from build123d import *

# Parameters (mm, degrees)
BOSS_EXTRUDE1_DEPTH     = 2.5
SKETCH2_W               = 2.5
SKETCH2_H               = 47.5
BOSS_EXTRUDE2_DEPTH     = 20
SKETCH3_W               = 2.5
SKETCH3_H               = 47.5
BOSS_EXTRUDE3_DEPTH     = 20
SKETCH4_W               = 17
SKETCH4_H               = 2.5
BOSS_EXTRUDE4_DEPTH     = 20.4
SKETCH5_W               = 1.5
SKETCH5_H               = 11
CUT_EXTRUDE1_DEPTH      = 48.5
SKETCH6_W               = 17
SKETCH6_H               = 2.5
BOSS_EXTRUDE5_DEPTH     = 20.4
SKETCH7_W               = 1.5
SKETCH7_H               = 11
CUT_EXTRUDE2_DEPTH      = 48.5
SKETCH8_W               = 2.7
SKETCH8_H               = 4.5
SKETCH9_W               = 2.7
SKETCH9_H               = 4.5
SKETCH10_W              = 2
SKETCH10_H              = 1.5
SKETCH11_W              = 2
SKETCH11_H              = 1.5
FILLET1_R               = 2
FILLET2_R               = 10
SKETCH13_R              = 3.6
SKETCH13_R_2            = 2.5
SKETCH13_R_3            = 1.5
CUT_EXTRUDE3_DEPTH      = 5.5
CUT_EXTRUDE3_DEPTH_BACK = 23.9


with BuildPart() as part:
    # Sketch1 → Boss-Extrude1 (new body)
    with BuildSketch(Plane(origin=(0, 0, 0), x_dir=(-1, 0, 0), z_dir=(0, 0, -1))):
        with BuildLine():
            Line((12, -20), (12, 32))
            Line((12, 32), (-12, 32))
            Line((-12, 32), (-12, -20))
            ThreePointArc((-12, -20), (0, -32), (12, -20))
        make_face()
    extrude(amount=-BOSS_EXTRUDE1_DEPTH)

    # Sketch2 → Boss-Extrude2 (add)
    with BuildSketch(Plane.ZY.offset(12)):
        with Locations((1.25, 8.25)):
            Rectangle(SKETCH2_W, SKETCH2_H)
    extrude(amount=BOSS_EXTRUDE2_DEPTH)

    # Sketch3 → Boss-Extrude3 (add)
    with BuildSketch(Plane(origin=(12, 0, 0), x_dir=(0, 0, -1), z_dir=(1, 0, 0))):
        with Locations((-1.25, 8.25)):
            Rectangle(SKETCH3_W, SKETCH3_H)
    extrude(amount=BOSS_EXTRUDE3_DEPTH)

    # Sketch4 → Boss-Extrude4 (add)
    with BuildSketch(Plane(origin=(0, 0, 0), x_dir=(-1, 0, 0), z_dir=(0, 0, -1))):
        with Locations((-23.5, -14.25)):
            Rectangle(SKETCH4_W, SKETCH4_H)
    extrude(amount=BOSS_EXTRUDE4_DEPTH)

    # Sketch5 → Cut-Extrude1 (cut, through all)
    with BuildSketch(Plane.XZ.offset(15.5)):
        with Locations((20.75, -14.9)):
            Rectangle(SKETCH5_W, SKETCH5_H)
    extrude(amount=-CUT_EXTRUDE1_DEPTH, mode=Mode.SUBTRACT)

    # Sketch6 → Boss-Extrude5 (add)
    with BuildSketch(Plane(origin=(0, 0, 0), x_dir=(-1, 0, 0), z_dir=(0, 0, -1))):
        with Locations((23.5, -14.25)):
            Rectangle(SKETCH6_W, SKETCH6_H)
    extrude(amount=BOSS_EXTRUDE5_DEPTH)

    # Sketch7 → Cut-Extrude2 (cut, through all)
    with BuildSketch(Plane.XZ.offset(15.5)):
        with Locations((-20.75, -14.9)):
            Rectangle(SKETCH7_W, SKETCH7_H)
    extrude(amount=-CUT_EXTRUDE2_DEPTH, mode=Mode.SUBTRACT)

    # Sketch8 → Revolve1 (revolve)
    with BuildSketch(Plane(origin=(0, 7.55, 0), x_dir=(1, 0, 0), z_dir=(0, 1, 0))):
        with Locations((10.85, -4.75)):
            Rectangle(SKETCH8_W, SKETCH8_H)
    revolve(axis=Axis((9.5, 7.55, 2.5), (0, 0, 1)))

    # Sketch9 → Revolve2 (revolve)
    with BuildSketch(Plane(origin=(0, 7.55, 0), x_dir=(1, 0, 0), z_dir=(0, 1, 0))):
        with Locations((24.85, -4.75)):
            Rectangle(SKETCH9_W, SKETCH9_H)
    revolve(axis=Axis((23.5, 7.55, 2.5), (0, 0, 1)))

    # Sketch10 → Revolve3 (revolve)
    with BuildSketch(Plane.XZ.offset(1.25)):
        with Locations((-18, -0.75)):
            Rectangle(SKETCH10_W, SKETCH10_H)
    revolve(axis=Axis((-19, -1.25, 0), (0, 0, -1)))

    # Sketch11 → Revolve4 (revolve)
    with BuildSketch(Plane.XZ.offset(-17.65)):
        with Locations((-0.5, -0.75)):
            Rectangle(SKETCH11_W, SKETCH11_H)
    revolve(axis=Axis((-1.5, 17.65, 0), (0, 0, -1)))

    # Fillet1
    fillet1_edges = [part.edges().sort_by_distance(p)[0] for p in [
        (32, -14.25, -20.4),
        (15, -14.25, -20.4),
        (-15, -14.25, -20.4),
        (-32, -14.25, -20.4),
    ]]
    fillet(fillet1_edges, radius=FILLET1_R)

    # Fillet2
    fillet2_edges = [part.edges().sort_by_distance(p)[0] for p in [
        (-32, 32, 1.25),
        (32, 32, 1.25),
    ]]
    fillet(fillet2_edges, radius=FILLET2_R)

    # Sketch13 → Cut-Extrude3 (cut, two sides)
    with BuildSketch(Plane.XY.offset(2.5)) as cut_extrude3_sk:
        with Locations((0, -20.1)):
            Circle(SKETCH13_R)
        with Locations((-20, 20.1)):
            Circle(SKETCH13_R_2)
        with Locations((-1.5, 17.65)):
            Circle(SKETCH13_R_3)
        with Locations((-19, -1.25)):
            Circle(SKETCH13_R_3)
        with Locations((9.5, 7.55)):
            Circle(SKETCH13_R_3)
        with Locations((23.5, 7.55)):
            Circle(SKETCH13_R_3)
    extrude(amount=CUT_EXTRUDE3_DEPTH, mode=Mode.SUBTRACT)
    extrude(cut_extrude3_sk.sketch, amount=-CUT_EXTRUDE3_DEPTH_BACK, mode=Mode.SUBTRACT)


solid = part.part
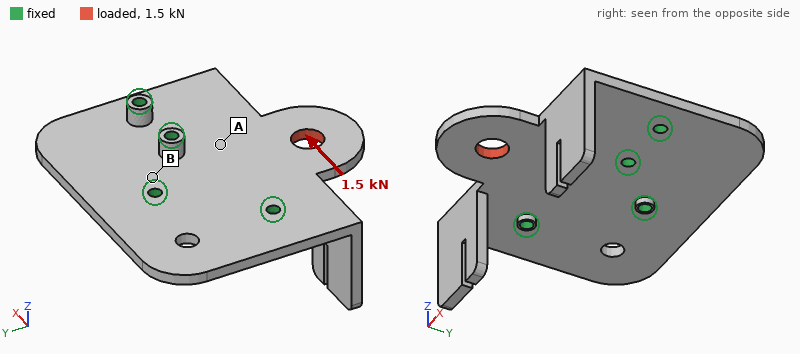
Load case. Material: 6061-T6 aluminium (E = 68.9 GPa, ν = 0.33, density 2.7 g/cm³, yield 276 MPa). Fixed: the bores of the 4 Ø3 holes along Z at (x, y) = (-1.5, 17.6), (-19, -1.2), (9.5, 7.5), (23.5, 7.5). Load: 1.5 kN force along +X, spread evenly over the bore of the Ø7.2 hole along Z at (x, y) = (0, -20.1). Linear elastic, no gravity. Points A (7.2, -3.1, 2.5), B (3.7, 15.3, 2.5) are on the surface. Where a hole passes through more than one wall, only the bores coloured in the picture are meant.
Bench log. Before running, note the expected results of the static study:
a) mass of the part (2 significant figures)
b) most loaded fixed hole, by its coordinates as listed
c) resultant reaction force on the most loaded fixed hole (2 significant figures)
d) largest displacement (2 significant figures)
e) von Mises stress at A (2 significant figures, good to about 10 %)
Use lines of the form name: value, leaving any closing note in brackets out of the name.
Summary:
mass of the part: 27 g
most loaded fixed hole, by its coordinates as listed: (-19, -1.2)
resultant reaction force on the most loaded fixed hole: 1.2 kN
largest displacement: 29 µm
von Mises stress at A: 17 MPa
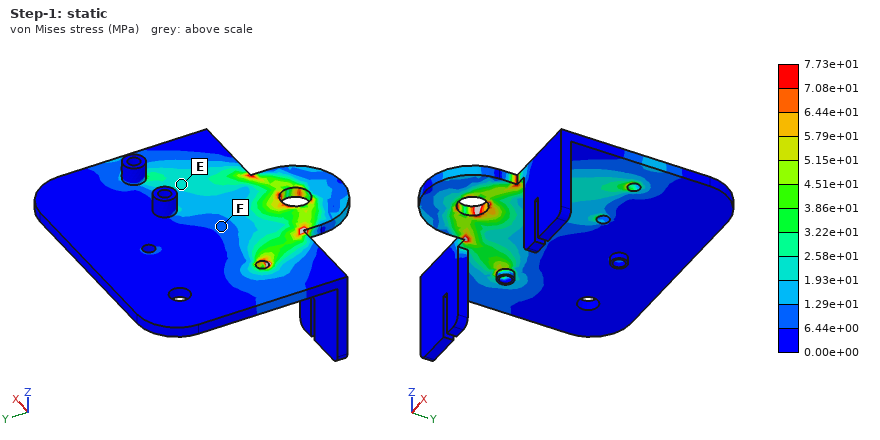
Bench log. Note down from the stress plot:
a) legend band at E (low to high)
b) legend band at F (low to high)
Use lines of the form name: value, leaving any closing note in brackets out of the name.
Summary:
legend band at E: 1.93e+01 to 2.58e+01 MPa
legend band at F: 6.44e+00 to 1.29e+01 MPa
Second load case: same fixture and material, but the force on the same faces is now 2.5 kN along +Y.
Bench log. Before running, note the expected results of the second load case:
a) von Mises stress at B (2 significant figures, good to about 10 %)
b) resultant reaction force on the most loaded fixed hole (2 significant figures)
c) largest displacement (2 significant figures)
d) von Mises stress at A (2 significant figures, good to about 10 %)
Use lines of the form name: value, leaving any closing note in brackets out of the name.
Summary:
von Mises stress at B: 5.9 MPa
resultant reaction force on the most loaded fixed hole: 840 N
largest displacement: 20 µm
von Mises stress at A: 34 MPa
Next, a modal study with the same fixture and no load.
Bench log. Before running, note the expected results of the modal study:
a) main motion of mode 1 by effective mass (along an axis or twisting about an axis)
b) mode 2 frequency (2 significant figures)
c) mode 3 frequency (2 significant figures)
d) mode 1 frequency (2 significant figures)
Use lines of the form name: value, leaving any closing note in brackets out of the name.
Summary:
main motion of mode 1 by effective mass: along Z
mode 2 frequency: 2500 Hz
mode 3 frequency: 2900 Hz
mode 1 frequency: 1900 Hz
